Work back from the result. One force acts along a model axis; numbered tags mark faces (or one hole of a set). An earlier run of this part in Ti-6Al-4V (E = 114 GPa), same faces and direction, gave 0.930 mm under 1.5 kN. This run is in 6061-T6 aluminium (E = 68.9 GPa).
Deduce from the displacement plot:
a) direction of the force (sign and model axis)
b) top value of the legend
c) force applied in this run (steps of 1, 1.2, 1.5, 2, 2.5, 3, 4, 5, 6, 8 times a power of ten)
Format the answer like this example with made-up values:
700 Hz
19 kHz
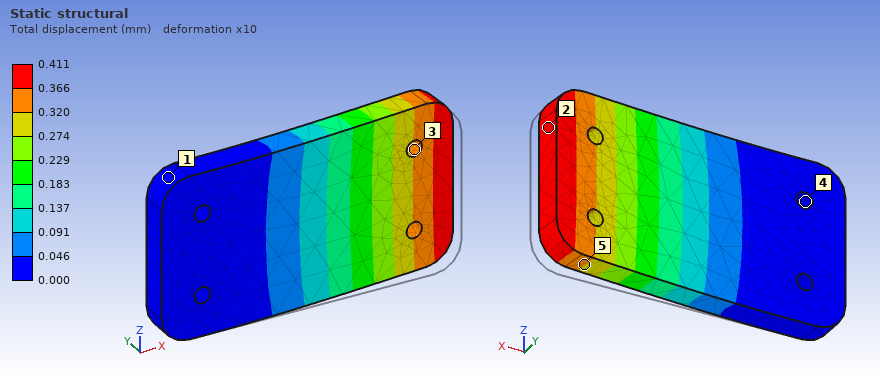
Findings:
+Y
0.411 mm
400 N
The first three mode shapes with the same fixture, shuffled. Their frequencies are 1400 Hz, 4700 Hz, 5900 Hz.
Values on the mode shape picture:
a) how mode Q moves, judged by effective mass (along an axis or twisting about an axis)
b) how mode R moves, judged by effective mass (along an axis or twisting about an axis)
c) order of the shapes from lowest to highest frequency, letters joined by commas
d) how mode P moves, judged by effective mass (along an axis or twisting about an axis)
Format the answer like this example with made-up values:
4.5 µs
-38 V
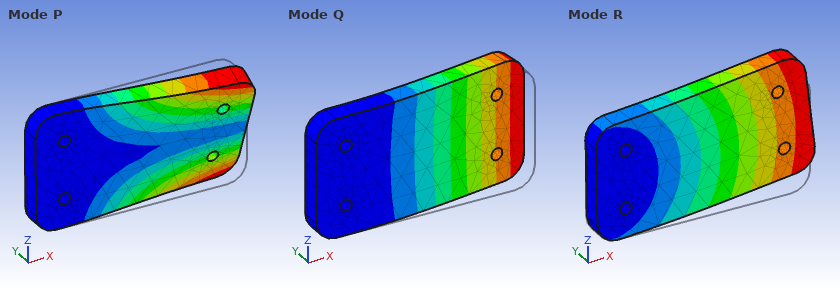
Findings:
along Y
along Z
Q, P, R
twisting about X
